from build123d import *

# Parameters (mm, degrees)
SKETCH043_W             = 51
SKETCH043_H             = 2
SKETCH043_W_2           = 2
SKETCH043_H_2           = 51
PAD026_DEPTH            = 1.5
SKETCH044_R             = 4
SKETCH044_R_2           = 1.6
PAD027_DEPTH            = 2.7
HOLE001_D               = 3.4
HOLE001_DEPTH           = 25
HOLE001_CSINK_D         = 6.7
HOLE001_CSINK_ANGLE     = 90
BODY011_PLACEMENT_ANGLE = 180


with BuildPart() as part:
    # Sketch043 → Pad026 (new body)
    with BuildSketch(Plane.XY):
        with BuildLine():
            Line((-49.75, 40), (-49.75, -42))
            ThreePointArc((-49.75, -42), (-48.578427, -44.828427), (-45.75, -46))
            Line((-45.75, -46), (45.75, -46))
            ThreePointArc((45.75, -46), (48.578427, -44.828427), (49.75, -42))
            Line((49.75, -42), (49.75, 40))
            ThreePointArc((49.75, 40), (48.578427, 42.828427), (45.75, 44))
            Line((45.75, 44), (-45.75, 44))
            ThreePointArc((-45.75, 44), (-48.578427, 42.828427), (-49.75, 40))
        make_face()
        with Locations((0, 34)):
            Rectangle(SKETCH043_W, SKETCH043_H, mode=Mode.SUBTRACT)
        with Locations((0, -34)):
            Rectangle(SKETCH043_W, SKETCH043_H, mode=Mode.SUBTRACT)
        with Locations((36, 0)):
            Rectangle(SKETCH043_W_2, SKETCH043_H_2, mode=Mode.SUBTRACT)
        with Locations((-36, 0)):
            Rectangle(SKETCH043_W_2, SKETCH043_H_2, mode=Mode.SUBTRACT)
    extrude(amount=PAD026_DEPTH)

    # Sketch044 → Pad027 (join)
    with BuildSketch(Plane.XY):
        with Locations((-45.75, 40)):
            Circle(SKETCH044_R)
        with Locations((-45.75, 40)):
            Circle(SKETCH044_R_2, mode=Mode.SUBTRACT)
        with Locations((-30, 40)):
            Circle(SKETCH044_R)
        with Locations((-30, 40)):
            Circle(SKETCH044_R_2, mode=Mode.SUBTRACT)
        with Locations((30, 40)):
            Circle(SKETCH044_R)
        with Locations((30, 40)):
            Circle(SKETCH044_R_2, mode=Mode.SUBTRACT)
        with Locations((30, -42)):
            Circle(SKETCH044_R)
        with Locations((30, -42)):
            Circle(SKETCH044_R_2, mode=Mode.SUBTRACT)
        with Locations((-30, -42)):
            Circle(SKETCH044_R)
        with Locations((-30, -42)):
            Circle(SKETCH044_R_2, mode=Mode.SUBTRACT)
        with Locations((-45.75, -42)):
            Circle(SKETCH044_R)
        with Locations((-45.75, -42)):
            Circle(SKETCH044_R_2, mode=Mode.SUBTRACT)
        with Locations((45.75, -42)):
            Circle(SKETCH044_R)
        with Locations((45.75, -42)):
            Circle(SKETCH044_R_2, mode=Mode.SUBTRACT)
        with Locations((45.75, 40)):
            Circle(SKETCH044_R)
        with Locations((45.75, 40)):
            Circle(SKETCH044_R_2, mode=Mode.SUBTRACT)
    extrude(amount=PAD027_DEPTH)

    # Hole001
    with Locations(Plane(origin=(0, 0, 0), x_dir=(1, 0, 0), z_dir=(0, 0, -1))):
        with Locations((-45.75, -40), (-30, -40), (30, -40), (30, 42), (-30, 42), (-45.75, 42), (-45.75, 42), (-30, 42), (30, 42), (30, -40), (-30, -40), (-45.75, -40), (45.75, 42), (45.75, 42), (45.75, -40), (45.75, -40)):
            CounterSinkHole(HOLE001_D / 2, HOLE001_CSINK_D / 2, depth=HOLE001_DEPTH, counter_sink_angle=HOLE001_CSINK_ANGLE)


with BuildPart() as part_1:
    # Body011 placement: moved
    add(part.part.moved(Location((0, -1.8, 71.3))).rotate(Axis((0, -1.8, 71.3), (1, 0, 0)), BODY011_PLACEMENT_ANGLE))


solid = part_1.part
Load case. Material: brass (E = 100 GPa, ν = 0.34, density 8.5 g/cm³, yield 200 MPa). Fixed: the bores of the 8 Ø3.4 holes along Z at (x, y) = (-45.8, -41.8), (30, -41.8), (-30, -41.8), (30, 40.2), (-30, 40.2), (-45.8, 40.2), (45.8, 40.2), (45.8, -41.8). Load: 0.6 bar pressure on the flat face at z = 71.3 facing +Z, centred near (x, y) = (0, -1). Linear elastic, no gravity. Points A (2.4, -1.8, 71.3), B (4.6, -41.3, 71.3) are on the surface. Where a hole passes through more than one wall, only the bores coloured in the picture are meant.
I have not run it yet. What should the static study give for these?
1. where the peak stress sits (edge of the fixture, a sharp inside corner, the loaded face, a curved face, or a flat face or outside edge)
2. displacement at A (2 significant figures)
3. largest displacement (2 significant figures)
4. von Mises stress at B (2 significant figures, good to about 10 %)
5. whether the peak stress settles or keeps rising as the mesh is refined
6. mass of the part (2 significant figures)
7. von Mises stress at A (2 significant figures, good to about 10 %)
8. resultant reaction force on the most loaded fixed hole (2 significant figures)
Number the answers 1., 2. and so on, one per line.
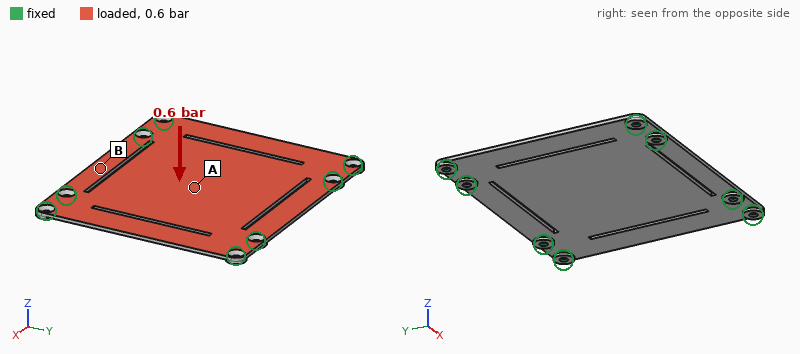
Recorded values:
1. edge of the fixture
2. 0.41 mm
3. 0.41 mm
4. 18 MPa
5. keeps rising
6. 110 g
7. 49 MPa
8. 220 N
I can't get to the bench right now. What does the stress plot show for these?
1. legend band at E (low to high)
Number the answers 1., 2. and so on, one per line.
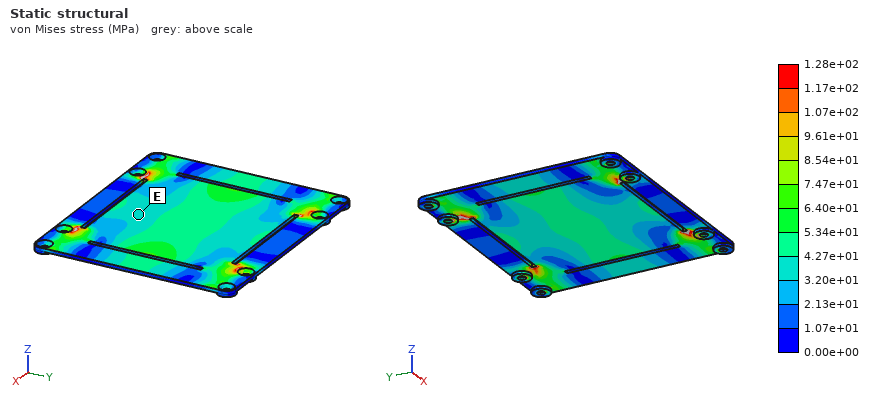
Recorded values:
1. 3.20e+01 to 4.27e+01 MPa
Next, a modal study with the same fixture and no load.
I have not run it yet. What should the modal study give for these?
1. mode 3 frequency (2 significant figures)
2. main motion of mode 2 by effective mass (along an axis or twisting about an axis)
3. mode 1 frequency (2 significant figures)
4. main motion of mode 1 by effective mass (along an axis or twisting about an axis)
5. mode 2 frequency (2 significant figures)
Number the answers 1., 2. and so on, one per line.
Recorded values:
1. 1000 Hz
2. twisting about Y
3. 640 Hz
4. along Z
5. 930 Hz
